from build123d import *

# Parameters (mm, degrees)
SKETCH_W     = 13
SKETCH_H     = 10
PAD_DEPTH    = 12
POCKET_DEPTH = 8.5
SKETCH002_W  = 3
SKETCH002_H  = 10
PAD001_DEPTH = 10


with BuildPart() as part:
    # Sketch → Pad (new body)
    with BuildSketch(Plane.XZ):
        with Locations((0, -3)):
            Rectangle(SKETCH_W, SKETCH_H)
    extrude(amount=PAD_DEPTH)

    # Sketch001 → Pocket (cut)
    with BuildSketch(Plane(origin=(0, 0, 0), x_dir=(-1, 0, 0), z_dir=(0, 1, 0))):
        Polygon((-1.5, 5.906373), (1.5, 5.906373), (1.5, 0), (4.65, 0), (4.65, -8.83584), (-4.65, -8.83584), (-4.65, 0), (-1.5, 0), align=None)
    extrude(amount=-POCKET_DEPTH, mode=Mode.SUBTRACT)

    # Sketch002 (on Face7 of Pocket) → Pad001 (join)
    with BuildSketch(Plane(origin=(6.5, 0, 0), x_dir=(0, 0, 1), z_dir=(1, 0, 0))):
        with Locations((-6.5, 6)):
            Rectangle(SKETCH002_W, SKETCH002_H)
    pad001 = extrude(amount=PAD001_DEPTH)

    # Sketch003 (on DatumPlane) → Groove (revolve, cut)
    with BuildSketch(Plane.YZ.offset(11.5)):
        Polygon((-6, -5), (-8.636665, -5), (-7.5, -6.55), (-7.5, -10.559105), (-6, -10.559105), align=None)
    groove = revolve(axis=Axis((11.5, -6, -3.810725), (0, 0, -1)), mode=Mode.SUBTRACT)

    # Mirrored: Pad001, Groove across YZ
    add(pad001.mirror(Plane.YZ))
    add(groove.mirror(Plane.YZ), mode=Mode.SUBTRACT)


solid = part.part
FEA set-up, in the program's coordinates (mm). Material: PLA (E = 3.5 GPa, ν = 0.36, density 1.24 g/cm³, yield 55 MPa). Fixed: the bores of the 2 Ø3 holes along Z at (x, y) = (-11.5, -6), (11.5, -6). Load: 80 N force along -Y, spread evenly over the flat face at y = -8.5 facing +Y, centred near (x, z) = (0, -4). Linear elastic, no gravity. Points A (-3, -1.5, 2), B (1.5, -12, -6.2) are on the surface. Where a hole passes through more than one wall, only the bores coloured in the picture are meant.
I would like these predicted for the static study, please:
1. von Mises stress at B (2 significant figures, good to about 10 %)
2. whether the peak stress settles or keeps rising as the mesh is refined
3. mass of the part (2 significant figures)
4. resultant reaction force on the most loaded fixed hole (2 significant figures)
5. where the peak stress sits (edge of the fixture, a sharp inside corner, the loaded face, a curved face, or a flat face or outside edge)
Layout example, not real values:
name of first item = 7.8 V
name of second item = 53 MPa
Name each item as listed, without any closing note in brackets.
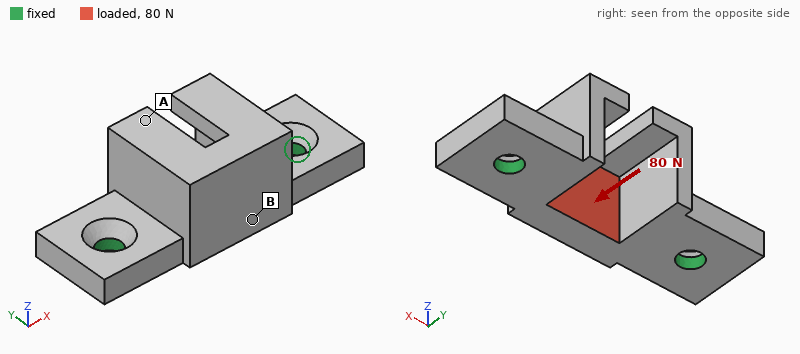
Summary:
von Mises stress at B = 6.2 MPa
whether the peak stress settles or keeps rising as the mesh is refined = keeps rising
mass of the part = 1.8 g
resultant reaction force on the most loaded fixed hole = 51 N
where the peak stress sits = edge of the fixture
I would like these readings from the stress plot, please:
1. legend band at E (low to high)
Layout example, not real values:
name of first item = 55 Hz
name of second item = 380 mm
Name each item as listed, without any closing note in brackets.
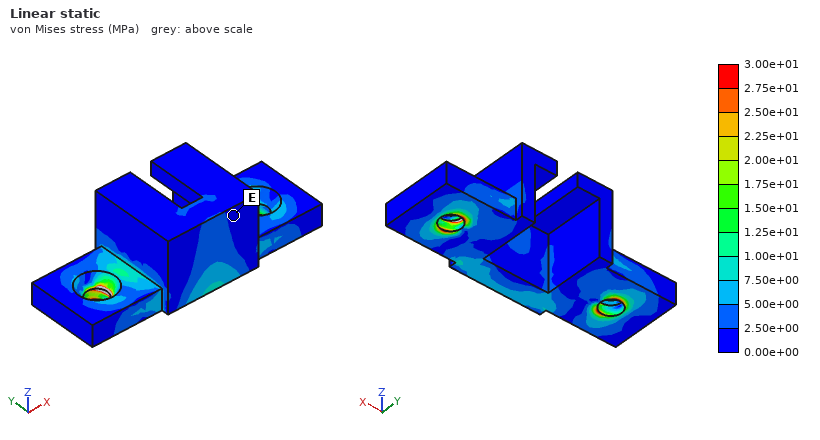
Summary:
legend band at E = 0.00e+00 to 2.50e+00 MPa
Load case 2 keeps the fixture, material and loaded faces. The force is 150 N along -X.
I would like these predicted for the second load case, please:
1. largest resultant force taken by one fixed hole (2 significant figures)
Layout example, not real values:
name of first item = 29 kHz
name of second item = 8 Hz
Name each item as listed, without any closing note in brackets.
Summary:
largest resultant force taken by one fixed hole = 79 N
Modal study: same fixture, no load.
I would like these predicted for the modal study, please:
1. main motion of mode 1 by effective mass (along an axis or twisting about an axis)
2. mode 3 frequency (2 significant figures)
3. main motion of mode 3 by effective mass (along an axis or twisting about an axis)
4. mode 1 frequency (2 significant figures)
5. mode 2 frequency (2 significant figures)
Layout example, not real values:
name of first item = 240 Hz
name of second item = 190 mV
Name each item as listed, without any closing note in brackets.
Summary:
main motion of mode 1 by effective mass = along Y
mode 3 frequency = 6900 Hz
main motion of mode 3 by effective mass = along Z
mode 1 frequency = 3600 Hz
mode 2 frequency = 6400 Hz
